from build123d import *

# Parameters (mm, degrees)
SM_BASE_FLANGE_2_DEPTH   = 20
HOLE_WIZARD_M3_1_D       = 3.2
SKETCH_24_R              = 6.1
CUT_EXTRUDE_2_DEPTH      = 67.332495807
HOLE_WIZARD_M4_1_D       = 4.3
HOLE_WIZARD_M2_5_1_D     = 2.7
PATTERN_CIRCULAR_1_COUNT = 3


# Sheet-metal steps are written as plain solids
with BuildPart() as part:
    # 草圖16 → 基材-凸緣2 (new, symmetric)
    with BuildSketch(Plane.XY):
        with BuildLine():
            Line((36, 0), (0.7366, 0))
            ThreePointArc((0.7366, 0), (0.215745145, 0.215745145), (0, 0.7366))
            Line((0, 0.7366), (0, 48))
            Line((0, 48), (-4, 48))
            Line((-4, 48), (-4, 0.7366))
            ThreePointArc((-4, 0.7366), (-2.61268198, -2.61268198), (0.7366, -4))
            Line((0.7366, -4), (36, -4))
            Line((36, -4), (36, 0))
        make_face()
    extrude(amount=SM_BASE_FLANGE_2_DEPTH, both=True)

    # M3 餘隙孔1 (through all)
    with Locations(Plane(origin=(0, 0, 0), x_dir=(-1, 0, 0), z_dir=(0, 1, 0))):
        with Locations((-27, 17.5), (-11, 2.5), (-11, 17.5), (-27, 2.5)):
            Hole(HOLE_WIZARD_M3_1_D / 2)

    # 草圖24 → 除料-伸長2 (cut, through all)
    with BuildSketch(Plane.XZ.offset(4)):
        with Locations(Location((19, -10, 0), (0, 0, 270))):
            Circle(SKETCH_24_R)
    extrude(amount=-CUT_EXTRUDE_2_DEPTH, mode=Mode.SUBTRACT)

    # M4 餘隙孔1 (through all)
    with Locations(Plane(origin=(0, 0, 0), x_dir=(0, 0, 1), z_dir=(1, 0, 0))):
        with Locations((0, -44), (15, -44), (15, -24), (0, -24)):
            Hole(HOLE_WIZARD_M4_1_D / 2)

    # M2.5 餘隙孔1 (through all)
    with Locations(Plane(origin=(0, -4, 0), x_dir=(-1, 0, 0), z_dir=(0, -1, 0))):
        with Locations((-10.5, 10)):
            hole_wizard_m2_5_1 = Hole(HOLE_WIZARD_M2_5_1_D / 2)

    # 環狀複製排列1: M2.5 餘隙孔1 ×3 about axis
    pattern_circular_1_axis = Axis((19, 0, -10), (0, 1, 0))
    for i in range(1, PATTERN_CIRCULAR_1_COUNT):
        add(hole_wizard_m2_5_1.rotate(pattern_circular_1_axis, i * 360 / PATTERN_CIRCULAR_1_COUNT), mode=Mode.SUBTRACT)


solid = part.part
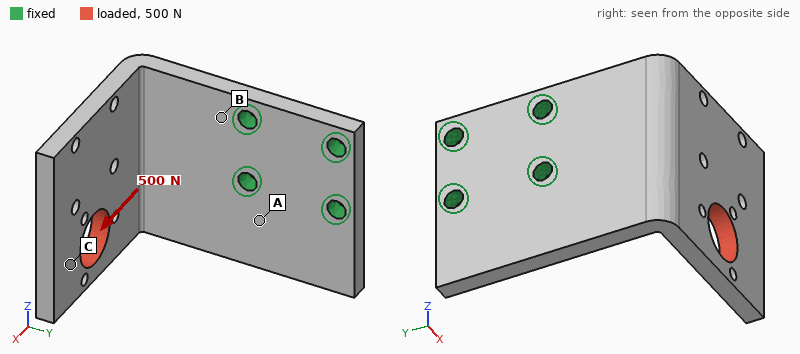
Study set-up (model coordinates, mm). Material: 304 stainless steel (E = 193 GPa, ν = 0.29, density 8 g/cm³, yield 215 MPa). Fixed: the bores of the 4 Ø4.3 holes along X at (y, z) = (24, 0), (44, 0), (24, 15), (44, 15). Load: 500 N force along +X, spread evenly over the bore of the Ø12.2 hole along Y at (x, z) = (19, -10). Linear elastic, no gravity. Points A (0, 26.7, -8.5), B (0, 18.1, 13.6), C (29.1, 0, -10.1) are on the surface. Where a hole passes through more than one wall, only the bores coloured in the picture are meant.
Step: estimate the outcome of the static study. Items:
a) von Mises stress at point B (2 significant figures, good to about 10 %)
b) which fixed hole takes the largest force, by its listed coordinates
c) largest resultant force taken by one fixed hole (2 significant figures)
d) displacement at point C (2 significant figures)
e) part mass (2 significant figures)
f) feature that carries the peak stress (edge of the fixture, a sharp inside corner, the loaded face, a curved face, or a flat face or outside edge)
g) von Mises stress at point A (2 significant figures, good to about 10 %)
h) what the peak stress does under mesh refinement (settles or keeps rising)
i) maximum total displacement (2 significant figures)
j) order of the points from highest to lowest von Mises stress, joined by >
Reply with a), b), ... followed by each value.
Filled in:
a) 80 MPa
b) (24, 0)
c) 820 N
d) 0.17 mm
e) 100 g
f) edge of the fixture
g) 66 MPa
h) keeps rising
i) 0.22 mm
j) B > A > C
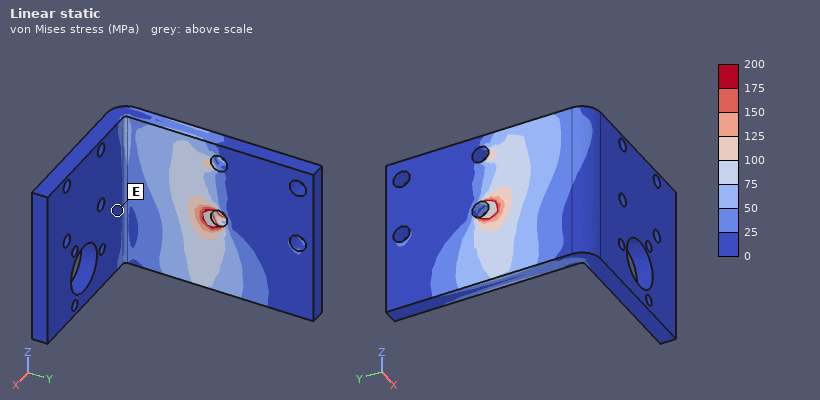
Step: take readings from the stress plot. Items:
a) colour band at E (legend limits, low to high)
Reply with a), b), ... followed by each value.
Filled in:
a) 0 to 25 MPa
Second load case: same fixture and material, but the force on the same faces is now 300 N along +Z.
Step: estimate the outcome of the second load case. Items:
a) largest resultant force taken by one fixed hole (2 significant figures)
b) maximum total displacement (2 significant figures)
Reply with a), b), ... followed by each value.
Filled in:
a) 470 N
b) 82 µm
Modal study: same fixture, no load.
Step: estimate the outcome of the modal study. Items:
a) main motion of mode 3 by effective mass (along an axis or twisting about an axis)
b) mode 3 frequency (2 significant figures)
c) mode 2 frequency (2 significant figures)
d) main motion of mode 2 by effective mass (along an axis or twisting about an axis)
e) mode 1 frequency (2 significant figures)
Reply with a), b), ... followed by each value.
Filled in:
a) along X
b) 3000 Hz
c) 1800 Hz
d) along Z
e) 1100 Hz
